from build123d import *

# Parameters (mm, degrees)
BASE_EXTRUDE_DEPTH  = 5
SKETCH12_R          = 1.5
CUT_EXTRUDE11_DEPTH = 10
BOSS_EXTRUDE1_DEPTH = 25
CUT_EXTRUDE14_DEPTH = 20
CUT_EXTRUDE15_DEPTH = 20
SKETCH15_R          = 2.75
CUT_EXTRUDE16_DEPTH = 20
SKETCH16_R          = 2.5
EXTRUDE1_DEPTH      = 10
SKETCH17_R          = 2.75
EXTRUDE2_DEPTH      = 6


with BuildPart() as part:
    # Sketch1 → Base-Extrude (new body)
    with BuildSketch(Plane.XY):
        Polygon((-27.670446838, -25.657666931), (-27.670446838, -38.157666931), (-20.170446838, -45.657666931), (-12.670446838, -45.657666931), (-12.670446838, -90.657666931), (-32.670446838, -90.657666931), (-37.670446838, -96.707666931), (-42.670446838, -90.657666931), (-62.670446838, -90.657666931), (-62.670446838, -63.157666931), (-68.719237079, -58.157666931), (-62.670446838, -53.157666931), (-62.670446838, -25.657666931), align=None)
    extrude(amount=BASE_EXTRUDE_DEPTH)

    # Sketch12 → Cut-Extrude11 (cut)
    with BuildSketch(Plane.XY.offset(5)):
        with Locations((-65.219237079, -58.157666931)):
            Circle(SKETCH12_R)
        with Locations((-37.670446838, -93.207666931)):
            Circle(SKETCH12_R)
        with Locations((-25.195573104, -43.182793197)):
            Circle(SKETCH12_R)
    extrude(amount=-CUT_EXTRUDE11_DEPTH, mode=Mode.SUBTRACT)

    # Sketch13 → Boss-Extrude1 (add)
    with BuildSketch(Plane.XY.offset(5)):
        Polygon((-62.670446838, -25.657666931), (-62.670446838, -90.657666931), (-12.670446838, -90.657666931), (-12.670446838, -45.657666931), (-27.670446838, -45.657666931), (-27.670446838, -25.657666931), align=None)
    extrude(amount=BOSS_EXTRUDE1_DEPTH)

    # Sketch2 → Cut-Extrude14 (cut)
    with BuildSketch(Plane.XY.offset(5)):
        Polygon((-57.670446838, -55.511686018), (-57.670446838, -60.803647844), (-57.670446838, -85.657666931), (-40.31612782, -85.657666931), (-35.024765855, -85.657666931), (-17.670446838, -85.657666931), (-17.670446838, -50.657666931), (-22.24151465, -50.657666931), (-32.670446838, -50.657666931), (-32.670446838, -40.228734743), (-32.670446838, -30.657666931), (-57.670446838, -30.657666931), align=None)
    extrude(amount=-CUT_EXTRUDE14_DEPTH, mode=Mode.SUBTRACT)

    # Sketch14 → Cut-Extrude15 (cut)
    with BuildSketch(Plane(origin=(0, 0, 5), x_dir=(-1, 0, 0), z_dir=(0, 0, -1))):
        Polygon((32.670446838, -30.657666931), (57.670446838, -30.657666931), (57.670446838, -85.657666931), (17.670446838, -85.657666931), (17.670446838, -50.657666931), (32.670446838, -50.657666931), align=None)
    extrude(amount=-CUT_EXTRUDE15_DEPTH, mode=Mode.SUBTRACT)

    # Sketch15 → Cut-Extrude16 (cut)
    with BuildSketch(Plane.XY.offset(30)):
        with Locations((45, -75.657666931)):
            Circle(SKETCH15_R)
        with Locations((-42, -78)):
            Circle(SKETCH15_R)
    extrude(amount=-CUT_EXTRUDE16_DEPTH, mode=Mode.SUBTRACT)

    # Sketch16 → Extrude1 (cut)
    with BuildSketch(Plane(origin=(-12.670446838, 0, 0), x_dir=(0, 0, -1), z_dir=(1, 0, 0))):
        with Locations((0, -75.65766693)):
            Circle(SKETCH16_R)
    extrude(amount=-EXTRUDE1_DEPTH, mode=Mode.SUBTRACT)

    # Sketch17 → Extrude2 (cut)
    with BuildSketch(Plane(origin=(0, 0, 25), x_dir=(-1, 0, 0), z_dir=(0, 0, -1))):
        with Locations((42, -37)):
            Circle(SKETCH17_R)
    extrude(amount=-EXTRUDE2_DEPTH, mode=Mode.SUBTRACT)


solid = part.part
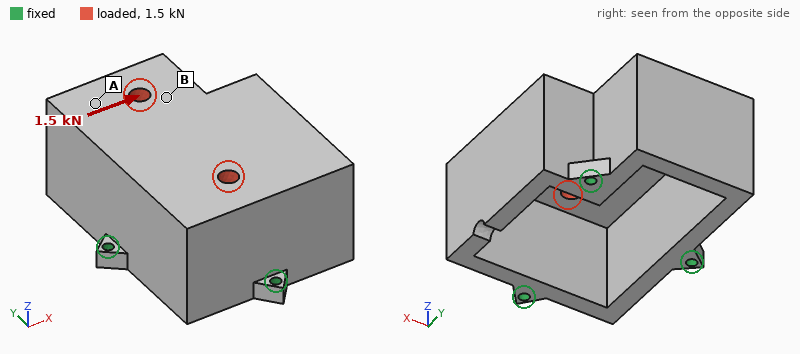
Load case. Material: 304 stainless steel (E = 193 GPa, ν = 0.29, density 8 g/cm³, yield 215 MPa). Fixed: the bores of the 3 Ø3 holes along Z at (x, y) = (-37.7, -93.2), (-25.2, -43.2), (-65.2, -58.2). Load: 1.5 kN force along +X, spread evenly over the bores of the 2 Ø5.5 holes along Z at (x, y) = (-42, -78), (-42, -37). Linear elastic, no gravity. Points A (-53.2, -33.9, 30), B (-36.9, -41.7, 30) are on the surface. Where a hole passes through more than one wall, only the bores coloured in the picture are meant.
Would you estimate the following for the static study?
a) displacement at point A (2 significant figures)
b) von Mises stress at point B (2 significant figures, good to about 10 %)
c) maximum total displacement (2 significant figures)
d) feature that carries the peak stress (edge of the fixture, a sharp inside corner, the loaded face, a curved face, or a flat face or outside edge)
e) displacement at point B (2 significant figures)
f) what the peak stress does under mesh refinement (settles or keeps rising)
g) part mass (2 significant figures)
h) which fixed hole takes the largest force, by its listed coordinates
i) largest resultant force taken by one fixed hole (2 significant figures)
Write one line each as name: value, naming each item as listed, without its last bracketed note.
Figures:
displacement at point A: 10 µm
von Mises stress at point B: 11 MPa
maximum total displacement: 12 µm
feature that carries the peak stress: edge of the fixture
displacement at point B: 10 µm
what the peak stress does under mesh refinement: keeps rising
part mass: 330 g
which fixed hole takes the largest force, by its listed coordinates: (-65.2, -58.2)
largest resultant force taken by one fixed hole: 1.1 kN
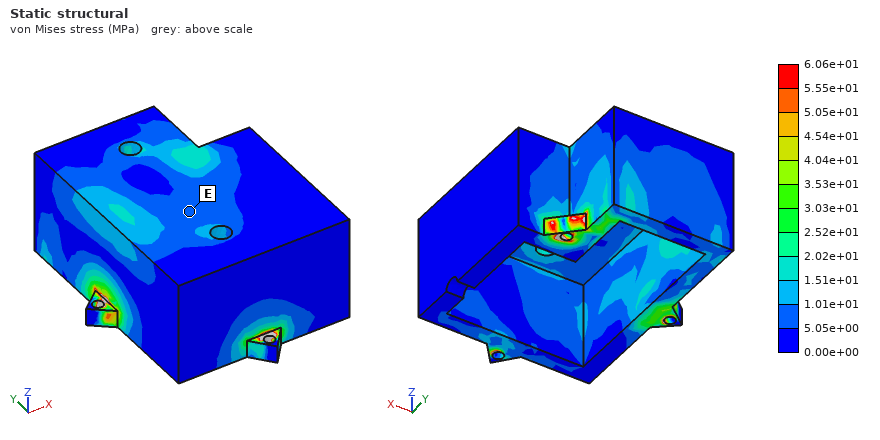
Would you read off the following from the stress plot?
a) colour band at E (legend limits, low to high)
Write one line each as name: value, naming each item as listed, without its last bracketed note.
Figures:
colour band at E: 5.05e+00 to 1.01e+01 MPa
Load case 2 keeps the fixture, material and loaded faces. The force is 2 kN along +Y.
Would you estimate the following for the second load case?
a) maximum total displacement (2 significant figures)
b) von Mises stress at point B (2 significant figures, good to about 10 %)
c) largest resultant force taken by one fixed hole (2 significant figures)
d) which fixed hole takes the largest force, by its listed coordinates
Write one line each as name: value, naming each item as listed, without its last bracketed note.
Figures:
maximum total displacement: 13 µm
von Mises stress at point B: 12 MPa
largest resultant force taken by one fixed hole: 1.2 kN
which fixed hole takes the largest force, by its listed coordinates: (-37.7, -93.2)
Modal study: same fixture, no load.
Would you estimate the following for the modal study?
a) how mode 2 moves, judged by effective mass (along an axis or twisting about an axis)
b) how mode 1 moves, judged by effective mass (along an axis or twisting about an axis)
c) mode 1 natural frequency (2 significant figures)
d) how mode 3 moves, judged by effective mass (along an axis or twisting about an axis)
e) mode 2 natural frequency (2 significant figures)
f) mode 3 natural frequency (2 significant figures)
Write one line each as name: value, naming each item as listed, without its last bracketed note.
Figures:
how mode 2 moves, judged by effective mass: along Y
how mode 1 moves, judged by effective mass: along X
mode 1 natural frequency: 4100 Hz
how mode 3 moves, judged by effective mass: twisting about Z
mode 2 natural frequency: 4800 Hz
mode 3 natural frequency: 6600 Hz
